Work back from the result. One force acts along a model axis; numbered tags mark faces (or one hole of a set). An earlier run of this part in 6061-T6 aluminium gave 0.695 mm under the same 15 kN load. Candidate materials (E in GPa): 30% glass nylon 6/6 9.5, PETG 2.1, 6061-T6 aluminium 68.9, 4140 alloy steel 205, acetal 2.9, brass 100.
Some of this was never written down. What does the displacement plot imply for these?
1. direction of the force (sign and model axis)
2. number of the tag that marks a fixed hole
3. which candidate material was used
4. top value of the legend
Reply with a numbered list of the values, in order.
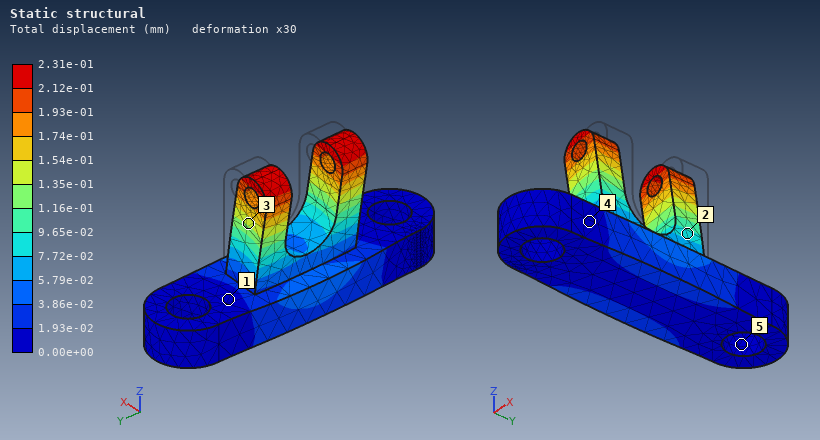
1. -X
2. 5
3. 4140 alloy steel
4. 2.31e-01 mm
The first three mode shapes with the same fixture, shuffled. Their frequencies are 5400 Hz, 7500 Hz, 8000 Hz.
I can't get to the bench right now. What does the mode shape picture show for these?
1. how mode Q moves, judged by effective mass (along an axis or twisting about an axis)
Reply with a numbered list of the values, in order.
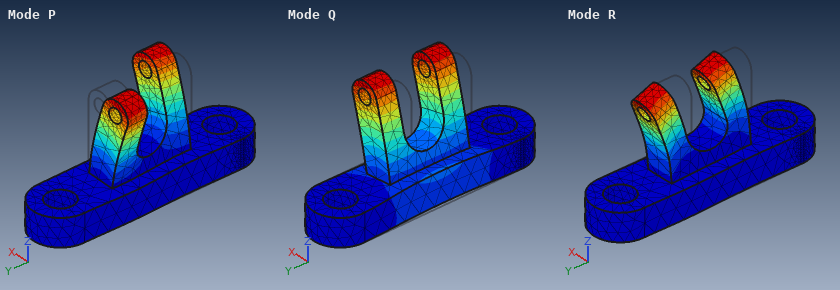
1. along X
